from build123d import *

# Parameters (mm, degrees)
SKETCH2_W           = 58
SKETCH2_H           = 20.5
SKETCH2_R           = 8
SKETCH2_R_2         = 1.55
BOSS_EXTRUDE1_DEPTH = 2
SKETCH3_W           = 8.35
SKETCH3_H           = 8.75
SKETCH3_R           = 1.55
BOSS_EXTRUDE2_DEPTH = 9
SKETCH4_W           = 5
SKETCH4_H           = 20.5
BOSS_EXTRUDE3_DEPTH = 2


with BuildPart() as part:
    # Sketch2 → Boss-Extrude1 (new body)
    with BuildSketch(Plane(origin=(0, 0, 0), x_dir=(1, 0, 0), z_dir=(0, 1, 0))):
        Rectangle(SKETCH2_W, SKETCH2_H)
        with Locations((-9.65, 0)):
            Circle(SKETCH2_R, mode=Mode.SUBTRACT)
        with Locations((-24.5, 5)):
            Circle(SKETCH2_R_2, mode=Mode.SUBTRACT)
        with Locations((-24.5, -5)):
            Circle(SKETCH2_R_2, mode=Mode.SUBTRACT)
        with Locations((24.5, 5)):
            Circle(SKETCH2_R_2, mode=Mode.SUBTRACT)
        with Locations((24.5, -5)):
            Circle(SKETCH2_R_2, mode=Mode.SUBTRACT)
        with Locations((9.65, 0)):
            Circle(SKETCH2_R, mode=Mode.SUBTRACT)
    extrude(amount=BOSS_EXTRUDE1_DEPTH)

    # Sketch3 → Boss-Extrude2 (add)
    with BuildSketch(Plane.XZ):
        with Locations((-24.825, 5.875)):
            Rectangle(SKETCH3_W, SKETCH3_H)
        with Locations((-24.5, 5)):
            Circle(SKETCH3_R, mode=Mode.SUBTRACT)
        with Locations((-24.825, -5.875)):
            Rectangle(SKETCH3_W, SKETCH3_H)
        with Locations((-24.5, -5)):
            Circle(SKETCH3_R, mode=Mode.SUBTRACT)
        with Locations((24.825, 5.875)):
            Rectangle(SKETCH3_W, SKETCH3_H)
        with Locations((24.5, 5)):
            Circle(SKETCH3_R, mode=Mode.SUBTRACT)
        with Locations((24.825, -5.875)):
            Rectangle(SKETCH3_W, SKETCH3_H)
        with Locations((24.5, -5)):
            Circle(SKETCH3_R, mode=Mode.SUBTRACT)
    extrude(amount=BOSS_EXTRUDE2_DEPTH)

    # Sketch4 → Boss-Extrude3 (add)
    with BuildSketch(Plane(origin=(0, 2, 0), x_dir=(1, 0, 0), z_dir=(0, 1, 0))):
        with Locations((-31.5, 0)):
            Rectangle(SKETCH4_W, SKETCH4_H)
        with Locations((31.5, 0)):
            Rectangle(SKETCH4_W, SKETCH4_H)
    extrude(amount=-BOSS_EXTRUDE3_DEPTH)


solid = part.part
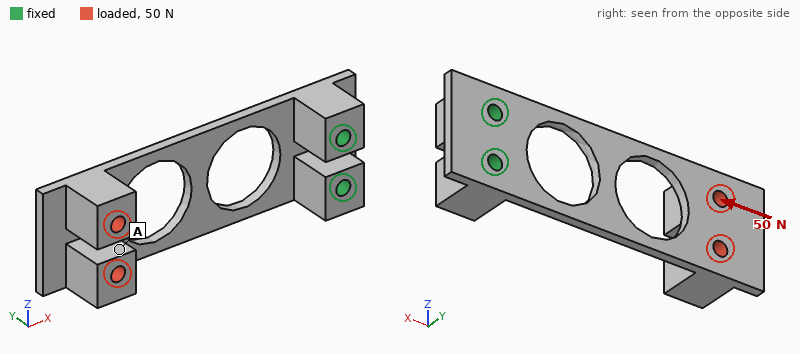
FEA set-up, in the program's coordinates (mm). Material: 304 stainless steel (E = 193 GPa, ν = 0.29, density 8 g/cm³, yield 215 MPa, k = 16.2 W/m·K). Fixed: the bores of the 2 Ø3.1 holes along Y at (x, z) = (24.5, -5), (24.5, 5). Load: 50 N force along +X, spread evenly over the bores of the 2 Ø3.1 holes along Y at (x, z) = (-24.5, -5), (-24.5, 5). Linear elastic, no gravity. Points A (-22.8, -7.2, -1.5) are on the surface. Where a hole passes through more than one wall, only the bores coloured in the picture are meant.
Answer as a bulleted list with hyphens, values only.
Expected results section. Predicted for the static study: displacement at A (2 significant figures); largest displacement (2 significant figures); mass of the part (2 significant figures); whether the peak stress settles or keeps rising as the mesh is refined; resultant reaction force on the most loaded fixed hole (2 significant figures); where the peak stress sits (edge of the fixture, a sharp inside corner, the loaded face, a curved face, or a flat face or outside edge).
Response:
- 0.25 mm
- 0.35 mm
- 34 g
- keeps rising
- 25 N
- a sharp inside corner
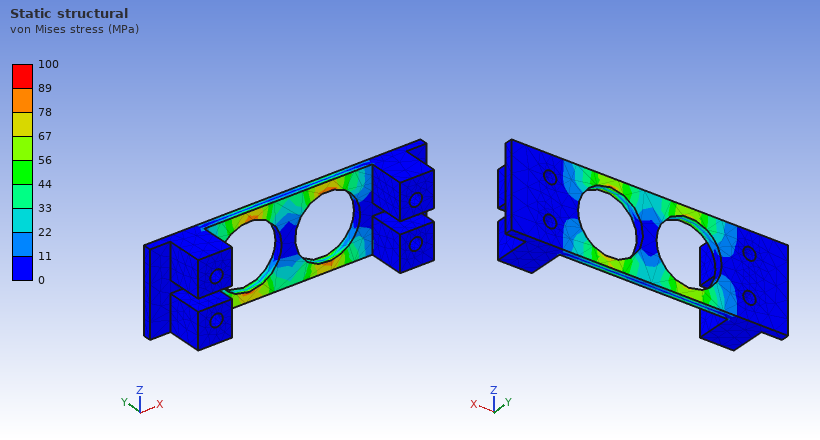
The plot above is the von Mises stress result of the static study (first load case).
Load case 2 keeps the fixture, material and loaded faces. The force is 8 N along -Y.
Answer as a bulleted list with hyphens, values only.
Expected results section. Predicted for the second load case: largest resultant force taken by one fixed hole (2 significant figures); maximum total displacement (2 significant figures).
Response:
- 4.3 N
- 0.35 mm
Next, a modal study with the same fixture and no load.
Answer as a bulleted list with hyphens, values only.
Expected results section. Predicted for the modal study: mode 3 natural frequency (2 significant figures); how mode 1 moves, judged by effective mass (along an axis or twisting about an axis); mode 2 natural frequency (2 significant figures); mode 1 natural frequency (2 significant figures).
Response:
- 2000 Hz
- along Y
- 1000 Hz
- 210 Hz
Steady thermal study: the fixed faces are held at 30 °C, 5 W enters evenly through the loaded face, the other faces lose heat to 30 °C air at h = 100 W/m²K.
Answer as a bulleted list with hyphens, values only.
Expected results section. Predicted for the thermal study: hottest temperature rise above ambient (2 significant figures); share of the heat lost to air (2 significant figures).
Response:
- 37 K
- 100 %
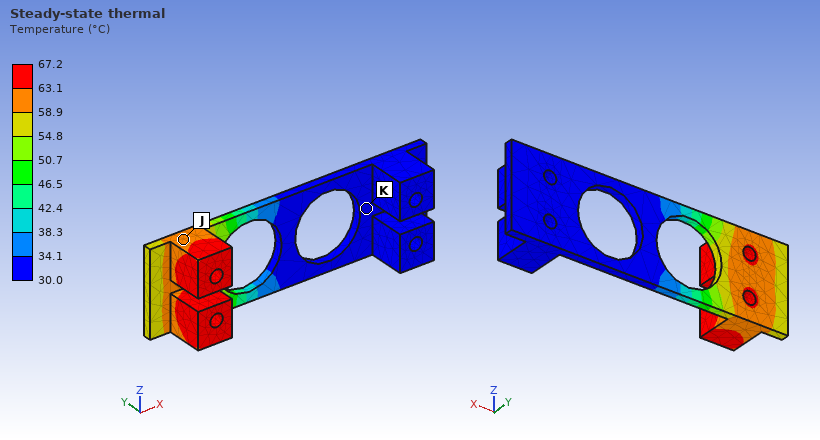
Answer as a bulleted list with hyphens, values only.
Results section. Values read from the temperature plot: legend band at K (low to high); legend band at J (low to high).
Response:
- 30.0 to 34.1 °C
- 58.9 to 63.1 °C
